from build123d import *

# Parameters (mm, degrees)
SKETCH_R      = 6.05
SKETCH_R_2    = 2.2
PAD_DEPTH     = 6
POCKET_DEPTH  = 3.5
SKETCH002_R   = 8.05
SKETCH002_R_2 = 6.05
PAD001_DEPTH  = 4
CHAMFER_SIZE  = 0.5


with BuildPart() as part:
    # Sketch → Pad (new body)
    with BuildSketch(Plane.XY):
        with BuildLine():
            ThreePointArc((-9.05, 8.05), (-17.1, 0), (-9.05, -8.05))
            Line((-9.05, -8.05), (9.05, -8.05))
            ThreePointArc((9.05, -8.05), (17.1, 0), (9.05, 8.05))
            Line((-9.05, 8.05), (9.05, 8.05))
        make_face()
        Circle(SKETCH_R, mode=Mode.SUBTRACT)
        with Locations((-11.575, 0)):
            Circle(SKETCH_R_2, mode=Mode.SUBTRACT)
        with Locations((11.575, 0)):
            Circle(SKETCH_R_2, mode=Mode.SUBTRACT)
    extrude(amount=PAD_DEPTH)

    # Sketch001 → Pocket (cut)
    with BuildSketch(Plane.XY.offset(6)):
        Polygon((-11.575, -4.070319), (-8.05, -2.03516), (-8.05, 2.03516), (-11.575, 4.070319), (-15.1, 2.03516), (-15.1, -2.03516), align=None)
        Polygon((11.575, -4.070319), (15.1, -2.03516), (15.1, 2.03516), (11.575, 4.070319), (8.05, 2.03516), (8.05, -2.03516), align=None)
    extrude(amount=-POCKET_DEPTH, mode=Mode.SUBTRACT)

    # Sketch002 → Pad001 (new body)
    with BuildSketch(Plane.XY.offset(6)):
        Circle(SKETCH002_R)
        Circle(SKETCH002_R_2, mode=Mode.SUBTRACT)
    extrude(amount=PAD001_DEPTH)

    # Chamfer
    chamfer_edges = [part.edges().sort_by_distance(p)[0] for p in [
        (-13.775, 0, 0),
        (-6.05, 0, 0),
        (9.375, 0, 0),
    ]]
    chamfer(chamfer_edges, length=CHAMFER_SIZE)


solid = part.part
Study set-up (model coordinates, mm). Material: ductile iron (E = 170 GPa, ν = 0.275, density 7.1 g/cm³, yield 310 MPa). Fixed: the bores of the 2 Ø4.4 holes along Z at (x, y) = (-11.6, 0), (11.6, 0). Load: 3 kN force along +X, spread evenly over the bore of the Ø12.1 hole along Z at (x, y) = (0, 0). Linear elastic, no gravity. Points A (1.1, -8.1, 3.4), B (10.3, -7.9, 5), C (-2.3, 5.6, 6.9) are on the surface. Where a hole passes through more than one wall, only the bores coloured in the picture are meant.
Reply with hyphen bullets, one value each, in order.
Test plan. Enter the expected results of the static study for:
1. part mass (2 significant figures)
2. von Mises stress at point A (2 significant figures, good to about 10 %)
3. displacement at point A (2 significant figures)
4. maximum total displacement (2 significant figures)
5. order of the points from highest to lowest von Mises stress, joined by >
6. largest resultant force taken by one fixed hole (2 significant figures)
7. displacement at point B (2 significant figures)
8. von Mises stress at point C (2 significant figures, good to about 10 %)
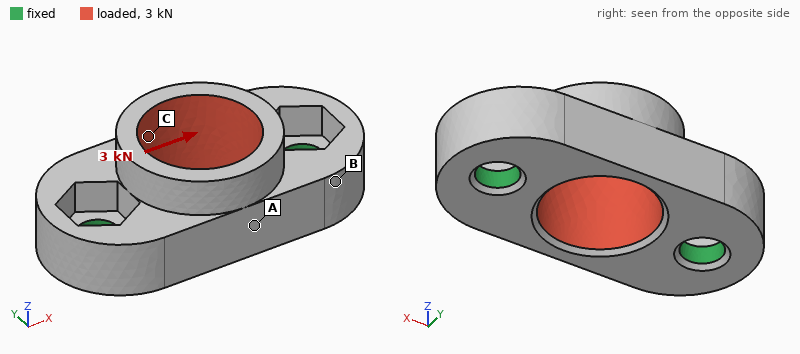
- 16 g
- 22 MPa
- 2.4 µm
- 5.3 µm
- C > A > B
- 1.6 kN
- 2.5 µm
- 40 MPa
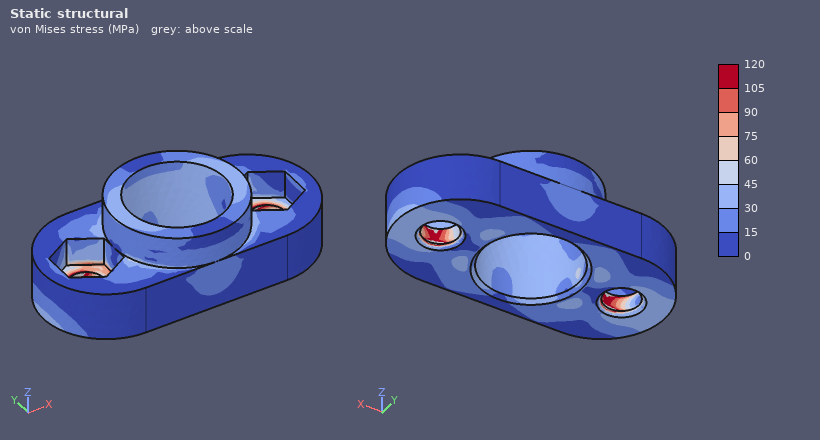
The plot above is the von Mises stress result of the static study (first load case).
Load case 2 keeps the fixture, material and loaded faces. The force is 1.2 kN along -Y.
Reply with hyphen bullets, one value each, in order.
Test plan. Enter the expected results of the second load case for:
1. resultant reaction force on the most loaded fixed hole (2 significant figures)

- 600 N
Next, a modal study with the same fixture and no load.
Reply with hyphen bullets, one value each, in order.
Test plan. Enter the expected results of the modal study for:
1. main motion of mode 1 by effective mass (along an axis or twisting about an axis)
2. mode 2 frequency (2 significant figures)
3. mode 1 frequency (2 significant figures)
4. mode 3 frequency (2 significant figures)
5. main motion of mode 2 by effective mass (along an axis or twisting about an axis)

- along Y
- 27 kHz
- 17 kHz
- 33 kHz
- along Z
